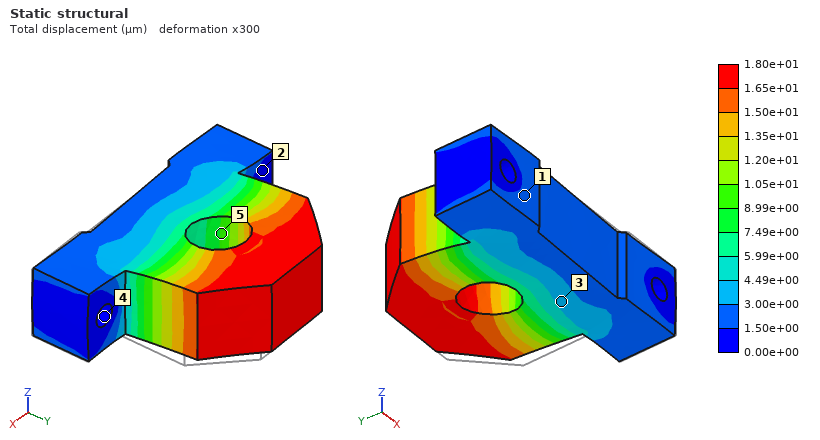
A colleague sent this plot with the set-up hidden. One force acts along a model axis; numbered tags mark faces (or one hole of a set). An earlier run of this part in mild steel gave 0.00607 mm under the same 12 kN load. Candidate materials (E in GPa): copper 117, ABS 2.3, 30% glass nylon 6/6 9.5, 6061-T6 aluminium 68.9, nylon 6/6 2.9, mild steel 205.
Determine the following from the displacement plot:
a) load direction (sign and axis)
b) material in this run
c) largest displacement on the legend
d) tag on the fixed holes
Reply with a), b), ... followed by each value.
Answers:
a) -X
b) 6061-T6 aluminium
c) 1.80e+01 µm
d) 4
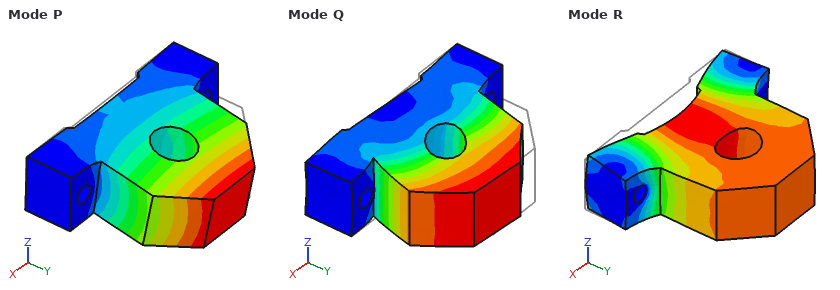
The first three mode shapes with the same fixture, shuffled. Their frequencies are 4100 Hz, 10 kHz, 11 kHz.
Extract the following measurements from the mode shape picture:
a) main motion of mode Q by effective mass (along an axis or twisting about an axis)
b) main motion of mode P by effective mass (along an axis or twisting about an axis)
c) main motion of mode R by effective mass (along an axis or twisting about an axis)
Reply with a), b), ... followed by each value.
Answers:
a) along X
b) along Z
c) along Y
